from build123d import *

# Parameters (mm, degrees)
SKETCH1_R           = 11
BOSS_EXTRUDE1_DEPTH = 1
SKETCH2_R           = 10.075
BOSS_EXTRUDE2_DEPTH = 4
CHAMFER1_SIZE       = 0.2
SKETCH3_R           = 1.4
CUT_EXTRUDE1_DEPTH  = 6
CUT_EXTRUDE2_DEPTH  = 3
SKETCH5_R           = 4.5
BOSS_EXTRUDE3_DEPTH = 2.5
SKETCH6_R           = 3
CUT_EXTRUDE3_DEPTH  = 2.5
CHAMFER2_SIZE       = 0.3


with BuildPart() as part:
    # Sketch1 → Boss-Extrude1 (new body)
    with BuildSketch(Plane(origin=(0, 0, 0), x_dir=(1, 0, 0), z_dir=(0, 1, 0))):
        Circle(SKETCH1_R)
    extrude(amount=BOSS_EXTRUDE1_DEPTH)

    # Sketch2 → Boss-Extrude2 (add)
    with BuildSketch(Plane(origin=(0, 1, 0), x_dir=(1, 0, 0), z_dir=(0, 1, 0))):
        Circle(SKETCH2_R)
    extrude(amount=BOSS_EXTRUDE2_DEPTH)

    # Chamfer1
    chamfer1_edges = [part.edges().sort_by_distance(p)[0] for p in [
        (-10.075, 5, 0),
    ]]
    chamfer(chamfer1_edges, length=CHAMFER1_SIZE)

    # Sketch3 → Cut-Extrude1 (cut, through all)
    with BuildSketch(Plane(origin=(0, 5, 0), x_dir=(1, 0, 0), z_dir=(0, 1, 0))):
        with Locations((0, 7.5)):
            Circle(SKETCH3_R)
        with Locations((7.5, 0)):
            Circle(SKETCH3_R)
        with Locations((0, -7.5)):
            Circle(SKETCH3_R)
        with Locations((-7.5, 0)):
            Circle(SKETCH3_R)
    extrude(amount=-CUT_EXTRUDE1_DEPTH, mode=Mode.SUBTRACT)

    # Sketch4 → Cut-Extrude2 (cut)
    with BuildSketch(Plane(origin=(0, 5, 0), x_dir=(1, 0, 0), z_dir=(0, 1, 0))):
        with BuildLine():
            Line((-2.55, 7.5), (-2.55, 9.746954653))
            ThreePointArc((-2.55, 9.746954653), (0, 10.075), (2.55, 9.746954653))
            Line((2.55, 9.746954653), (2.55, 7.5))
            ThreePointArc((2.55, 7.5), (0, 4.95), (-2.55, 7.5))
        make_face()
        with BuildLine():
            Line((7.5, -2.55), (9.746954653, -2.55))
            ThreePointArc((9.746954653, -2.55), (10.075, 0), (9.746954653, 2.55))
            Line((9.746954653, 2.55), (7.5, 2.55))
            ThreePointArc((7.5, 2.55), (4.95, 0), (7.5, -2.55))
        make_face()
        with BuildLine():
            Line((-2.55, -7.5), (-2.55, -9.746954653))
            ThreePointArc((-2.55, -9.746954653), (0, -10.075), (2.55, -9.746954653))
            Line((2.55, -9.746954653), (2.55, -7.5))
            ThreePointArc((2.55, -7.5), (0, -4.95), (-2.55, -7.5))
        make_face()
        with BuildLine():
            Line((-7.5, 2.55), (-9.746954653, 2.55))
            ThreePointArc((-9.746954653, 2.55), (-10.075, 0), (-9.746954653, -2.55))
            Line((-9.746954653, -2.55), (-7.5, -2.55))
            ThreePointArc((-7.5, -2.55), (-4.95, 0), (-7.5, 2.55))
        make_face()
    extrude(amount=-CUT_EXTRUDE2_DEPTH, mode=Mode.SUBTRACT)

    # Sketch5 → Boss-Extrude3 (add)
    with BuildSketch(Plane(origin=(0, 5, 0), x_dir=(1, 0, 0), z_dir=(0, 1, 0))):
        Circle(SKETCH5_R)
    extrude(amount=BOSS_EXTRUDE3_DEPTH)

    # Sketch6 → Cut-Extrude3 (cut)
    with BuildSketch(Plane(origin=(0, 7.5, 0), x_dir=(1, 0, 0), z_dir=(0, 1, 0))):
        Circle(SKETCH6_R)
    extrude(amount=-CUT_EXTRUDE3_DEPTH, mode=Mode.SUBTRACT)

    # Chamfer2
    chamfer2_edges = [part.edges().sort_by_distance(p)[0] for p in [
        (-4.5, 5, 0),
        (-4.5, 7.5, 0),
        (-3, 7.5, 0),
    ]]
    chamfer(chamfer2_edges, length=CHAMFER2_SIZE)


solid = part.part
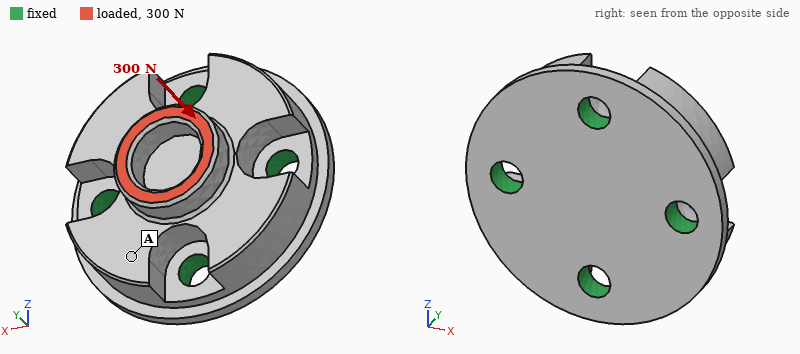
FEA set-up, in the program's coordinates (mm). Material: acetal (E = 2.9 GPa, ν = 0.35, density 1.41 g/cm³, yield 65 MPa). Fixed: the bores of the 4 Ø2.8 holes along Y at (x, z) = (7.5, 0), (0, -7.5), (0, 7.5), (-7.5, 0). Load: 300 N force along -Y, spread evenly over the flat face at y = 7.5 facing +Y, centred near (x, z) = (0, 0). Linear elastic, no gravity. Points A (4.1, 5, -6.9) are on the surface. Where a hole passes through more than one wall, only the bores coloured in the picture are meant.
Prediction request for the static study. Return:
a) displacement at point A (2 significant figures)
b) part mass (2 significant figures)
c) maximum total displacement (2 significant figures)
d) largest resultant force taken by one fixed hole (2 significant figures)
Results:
7.4 µm
2.0 g
25 µm
81 N
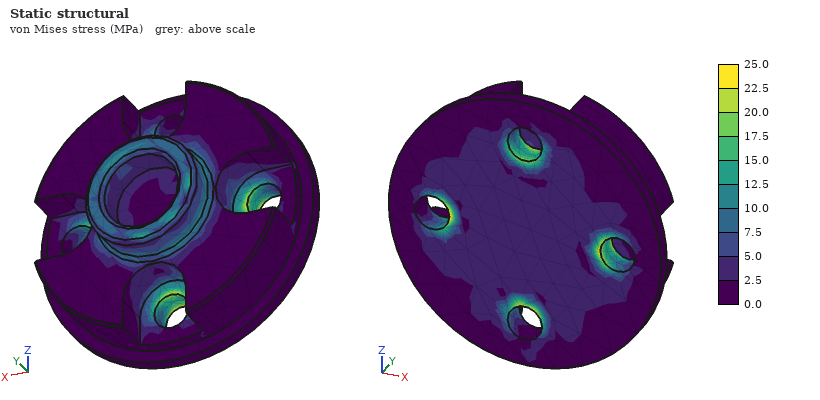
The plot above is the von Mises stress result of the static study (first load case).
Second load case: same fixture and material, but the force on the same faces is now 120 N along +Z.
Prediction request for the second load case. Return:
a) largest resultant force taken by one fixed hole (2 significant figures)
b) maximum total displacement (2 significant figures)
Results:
66 N
42 µm
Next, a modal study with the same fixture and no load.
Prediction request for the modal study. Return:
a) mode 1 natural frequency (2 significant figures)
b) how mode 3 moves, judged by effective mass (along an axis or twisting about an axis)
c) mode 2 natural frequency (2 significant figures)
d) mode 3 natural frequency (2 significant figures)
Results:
17 kHz
along Y
17 kHz
20 kHz
